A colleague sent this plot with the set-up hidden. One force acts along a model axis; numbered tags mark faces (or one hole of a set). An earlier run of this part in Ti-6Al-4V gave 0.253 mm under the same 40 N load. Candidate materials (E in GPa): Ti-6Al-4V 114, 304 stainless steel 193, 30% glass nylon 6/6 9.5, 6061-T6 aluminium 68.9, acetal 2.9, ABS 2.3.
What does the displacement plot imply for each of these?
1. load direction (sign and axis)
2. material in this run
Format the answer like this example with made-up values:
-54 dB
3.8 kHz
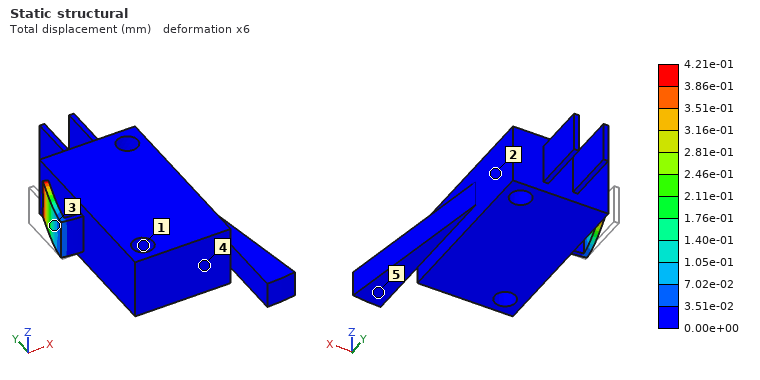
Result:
+X
6061-T6 aluminium
